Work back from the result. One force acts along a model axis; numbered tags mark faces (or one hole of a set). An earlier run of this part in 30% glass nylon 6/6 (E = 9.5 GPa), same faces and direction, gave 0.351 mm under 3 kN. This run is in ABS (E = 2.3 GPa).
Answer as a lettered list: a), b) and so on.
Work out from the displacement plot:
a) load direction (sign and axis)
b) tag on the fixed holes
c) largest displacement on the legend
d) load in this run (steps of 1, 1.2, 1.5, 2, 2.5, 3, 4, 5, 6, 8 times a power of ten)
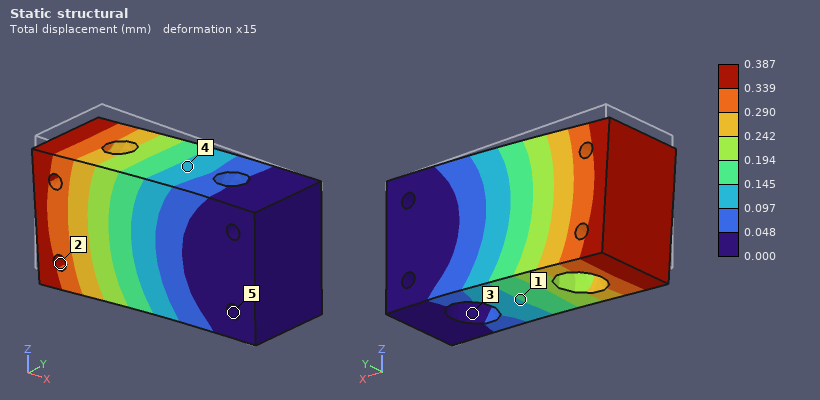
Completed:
a) -Z
b) 5
c) 0.387 mm
d) 800 N
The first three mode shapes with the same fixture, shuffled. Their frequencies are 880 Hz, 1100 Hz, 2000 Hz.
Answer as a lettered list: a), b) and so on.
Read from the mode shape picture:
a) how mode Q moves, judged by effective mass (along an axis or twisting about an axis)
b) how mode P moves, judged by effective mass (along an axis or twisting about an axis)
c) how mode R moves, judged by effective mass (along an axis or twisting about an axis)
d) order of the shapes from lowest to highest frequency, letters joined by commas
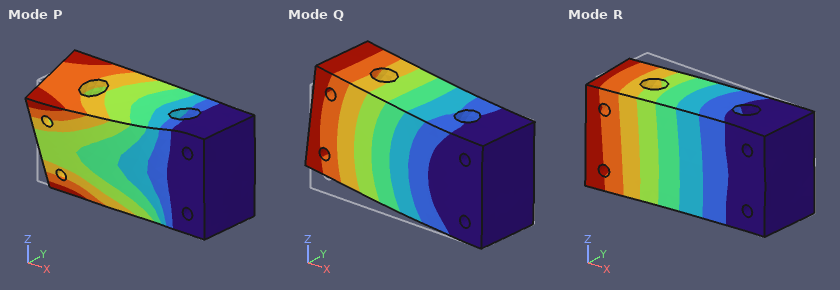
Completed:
a) along Z
b) twisting about X
c) along Y
d) R, Q, P
